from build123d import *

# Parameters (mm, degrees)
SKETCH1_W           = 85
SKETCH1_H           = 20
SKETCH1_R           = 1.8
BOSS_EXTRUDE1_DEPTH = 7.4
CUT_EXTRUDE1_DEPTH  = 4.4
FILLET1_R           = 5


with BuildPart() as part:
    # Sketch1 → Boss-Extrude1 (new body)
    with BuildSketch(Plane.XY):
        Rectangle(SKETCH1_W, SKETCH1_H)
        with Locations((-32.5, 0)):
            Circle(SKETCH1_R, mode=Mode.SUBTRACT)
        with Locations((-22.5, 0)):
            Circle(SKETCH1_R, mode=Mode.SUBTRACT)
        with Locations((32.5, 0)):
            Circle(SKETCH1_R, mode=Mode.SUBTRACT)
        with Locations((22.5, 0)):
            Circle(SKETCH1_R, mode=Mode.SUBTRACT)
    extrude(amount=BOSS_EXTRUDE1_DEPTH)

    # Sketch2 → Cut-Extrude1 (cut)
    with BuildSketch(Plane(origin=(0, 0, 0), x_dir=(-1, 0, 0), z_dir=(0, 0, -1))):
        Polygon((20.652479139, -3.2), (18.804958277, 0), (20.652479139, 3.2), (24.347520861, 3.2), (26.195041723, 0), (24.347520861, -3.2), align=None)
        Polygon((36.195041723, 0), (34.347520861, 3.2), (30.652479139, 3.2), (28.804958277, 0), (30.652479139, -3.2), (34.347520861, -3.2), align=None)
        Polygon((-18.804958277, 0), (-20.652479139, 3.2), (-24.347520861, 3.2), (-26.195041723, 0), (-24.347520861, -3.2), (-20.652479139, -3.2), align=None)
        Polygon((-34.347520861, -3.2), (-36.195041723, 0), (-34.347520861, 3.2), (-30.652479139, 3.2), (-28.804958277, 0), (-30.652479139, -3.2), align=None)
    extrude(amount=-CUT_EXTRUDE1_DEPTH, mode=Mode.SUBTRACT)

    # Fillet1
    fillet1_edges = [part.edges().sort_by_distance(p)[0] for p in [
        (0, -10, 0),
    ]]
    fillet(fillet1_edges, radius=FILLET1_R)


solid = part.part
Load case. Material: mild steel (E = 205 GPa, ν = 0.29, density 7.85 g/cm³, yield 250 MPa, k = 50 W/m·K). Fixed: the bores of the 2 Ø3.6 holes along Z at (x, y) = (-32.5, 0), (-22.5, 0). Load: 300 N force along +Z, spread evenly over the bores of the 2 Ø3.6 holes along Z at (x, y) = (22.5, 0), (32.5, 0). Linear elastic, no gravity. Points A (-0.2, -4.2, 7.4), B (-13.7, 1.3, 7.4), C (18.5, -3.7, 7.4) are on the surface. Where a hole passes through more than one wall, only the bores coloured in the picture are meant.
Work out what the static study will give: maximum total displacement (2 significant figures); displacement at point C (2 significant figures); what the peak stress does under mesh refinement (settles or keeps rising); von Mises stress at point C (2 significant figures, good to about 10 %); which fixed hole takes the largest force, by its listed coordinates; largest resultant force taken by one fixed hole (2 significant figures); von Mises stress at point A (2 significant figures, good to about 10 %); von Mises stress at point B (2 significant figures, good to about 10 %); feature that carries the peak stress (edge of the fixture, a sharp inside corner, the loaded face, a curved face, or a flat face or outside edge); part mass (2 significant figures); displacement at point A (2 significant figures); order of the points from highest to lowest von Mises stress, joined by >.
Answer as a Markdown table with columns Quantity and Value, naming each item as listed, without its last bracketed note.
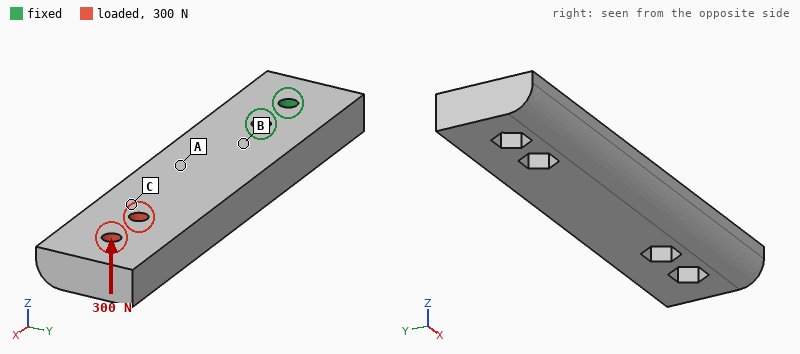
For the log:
| Quantity | Value |
|---|---|
| maximum total displacement | 0.19 mm |
| displacement at point C | 0.10 mm |
| what the peak stress does under mesh refinement | keeps rising |
| von Mises stress at point C | 19 MPa |
| which fixed hole takes the largest force, by its listed coordinates | (-22.5, 0) |
| largest resultant force taken by one fixed hole | 1.5 kN |
| von Mises stress at point A | 46 MPa |
| von Mises stress at point B | 68 MPa |
| feature that carries the peak stress | edge of the fixture |
| part mass | 89 g |
| displacement at point A | 0.042 mm |
| order of the points from highest to lowest von Mises stress, joined by > | B > A > C |
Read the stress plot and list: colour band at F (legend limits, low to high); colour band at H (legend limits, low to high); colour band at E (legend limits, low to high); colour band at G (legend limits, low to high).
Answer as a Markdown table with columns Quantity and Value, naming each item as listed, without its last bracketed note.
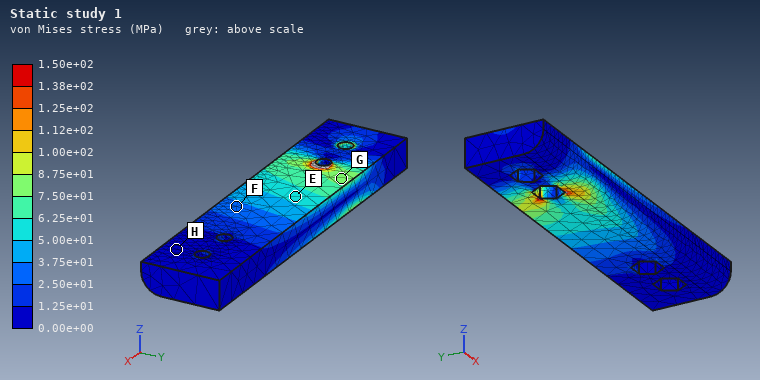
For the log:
| Quantity | Value |
|---|---|
| colour band at F | 2.50e+01 to 3.75e+01 MPa |
| colour band at H | 0.00e+00 to 1.25e+01 MPa |
| colour band at E | 5.00e+01 to 6.25e+01 MPa |
| colour band at G | 7.50e+01 to 8.75e+01 MPa |
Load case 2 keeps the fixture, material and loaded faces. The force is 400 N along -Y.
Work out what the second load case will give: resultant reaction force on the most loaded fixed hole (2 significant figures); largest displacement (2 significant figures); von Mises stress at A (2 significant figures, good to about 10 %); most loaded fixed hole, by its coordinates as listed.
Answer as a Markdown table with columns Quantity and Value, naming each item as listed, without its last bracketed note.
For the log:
| Quantity | Value |
|---|---|
| resultant reaction force on the most loaded fixed hole | 1.8 kN |
| largest displacement | 55 µm |
| von Mises stress at A | 15 MPa |
| most loaded fixed hole, by its coordinates as listed | (-22.5, 0) |
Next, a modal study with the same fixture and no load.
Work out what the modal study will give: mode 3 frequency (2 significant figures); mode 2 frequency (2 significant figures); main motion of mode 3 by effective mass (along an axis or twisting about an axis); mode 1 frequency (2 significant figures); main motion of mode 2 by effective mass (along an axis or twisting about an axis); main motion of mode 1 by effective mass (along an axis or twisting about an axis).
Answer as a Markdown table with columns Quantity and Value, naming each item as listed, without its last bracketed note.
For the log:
| Quantity | Value |
|---|---|
| mode 3 frequency | 6100 Hz |
| mode 2 frequency | 2600 Hz |
| main motion of mode 3 by effective mass | twisting about X |
| mode 1 frequency | 1200 Hz |
| main motion of mode 2 by effective mass | along Y |
| main motion of mode 1 by effective mass | along Z |
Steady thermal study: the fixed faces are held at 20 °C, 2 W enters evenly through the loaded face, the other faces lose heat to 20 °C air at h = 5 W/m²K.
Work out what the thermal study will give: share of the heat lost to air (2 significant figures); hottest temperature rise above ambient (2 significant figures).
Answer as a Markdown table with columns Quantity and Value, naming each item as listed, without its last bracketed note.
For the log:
| Quantity | Value |
|---|---|
| share of the heat lost to air | 9.3 % |
| hottest temperature rise above ambient | 16 K |
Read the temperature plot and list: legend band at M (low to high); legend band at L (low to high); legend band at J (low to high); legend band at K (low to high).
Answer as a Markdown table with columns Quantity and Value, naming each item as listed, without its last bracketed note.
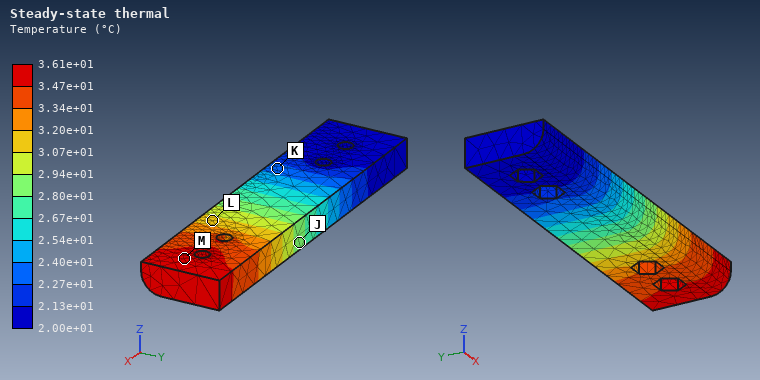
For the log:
| Quantity | Value |
|---|---|
| legend band at M | 3.47e+01 to 3.61e+01 °C |
| legend band at L | 3.07e+01 to 3.20e+01 °C |
| legend band at J | 2.80e+01 to 2.94e+01 °C |
| legend band at K | 2.27e+01 to 2.40e+01 °C |
